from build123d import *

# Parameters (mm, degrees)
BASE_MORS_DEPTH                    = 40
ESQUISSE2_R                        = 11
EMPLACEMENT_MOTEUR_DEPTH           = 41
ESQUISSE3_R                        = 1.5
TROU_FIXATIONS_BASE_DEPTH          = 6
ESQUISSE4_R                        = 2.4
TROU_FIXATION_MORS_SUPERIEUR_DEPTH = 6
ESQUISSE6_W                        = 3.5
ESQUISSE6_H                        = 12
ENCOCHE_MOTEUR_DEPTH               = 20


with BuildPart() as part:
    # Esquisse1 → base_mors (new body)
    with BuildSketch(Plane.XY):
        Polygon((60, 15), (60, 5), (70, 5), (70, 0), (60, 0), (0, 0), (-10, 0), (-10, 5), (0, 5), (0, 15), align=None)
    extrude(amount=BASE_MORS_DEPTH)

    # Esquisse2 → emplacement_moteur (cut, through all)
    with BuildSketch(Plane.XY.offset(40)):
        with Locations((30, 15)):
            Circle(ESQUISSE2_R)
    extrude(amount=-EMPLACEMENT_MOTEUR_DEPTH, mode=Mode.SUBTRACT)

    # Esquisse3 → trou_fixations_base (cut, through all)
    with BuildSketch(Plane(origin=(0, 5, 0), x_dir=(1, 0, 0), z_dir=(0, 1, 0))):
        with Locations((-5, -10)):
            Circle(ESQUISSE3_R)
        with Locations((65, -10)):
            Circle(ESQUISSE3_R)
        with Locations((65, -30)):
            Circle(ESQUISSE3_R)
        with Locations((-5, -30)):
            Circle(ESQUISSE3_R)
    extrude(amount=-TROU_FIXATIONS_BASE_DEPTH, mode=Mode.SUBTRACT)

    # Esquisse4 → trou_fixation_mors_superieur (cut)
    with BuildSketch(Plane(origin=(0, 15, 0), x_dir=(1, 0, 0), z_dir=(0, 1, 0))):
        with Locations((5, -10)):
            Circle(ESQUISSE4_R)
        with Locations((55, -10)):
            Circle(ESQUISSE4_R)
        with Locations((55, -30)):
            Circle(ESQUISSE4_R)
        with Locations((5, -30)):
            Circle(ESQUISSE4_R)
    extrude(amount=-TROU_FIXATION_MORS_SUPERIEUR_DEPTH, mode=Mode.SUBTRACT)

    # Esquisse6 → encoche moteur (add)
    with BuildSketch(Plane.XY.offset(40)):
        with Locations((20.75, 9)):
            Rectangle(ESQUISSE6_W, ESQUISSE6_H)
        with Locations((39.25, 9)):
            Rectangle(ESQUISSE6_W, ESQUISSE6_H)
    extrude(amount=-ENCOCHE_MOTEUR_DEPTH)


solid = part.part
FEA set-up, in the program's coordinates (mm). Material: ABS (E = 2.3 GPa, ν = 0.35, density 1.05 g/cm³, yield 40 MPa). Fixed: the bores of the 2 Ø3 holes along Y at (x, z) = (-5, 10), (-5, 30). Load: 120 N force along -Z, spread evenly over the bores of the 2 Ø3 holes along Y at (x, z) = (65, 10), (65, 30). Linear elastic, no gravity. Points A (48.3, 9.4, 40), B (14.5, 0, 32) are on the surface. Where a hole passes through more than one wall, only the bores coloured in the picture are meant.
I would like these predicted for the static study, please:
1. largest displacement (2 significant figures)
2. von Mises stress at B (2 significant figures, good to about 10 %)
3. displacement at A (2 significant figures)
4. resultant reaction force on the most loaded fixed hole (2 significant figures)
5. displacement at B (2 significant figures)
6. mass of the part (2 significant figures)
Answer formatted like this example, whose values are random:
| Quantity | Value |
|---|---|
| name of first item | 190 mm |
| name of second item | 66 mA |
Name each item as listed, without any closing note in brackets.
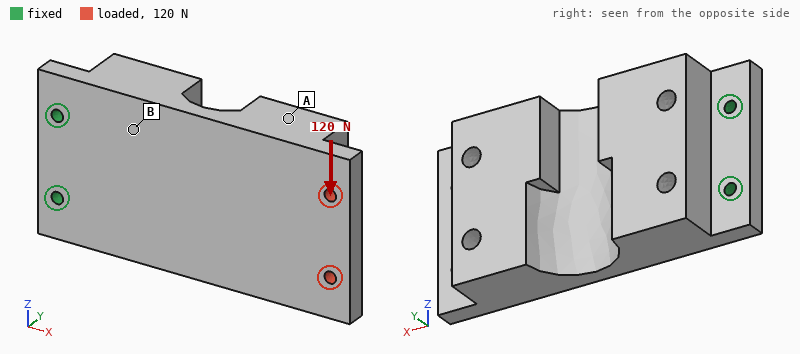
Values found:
| Quantity | Value |
|---|---|
| largest displacement | 0.43 mm |
| von Mises stress at B | 2.8 MPa |
| displacement at A | 0.28 mm |
| resultant reaction force on the most loaded fixed hole | 390 N |
| displacement at B | 0.090 mm |
| mass of the part | 34 g |
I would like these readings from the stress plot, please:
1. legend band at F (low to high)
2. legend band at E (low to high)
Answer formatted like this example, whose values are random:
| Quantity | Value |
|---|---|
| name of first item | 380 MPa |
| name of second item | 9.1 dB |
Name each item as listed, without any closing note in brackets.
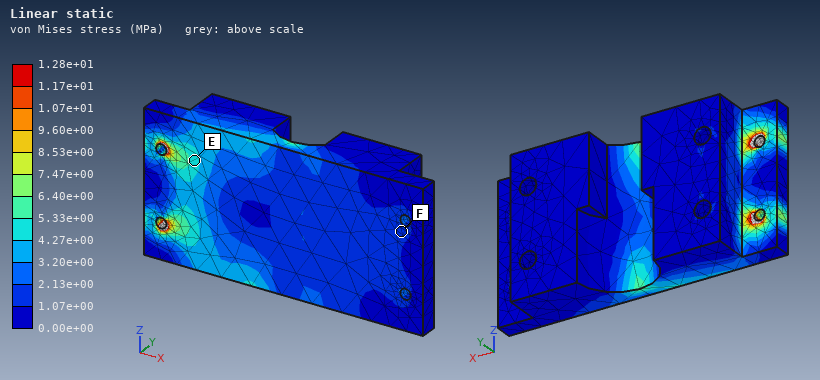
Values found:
| Quantity | Value |
|---|---|
| legend band at F | 1.07e+00 to 2.13e+00 MPa |
| legend band at E | 4.27e+00 to 5.33e+00 MPa |
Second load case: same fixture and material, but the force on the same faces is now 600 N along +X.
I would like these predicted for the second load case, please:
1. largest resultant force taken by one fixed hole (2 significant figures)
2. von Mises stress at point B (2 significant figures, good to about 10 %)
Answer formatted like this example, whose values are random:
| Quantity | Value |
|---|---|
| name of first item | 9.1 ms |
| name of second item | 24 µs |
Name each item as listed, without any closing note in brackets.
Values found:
| Quantity | Value |
|---|---|
| largest resultant force taken by one fixed hole | 300 N |
| von Mises stress at point B | 3.3 MPa |
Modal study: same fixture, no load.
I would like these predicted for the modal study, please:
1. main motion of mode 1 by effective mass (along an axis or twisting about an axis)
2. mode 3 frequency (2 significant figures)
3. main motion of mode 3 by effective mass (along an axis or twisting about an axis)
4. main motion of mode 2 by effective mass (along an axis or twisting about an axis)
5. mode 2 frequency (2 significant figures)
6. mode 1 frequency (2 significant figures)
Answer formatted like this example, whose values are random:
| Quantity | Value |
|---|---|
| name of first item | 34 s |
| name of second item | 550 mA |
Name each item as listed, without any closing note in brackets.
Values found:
| Quantity | Value |
|---|---|
| main motion of mode 1 by effective mass | along Y |
| mode 3 frequency | 1000 Hz |
| main motion of mode 3 by effective mass | along Y |
| main motion of mode 2 by effective mass | along Z |
| mode 2 frequency | 860 Hz |
| mode 1 frequency | 190 Hz |
